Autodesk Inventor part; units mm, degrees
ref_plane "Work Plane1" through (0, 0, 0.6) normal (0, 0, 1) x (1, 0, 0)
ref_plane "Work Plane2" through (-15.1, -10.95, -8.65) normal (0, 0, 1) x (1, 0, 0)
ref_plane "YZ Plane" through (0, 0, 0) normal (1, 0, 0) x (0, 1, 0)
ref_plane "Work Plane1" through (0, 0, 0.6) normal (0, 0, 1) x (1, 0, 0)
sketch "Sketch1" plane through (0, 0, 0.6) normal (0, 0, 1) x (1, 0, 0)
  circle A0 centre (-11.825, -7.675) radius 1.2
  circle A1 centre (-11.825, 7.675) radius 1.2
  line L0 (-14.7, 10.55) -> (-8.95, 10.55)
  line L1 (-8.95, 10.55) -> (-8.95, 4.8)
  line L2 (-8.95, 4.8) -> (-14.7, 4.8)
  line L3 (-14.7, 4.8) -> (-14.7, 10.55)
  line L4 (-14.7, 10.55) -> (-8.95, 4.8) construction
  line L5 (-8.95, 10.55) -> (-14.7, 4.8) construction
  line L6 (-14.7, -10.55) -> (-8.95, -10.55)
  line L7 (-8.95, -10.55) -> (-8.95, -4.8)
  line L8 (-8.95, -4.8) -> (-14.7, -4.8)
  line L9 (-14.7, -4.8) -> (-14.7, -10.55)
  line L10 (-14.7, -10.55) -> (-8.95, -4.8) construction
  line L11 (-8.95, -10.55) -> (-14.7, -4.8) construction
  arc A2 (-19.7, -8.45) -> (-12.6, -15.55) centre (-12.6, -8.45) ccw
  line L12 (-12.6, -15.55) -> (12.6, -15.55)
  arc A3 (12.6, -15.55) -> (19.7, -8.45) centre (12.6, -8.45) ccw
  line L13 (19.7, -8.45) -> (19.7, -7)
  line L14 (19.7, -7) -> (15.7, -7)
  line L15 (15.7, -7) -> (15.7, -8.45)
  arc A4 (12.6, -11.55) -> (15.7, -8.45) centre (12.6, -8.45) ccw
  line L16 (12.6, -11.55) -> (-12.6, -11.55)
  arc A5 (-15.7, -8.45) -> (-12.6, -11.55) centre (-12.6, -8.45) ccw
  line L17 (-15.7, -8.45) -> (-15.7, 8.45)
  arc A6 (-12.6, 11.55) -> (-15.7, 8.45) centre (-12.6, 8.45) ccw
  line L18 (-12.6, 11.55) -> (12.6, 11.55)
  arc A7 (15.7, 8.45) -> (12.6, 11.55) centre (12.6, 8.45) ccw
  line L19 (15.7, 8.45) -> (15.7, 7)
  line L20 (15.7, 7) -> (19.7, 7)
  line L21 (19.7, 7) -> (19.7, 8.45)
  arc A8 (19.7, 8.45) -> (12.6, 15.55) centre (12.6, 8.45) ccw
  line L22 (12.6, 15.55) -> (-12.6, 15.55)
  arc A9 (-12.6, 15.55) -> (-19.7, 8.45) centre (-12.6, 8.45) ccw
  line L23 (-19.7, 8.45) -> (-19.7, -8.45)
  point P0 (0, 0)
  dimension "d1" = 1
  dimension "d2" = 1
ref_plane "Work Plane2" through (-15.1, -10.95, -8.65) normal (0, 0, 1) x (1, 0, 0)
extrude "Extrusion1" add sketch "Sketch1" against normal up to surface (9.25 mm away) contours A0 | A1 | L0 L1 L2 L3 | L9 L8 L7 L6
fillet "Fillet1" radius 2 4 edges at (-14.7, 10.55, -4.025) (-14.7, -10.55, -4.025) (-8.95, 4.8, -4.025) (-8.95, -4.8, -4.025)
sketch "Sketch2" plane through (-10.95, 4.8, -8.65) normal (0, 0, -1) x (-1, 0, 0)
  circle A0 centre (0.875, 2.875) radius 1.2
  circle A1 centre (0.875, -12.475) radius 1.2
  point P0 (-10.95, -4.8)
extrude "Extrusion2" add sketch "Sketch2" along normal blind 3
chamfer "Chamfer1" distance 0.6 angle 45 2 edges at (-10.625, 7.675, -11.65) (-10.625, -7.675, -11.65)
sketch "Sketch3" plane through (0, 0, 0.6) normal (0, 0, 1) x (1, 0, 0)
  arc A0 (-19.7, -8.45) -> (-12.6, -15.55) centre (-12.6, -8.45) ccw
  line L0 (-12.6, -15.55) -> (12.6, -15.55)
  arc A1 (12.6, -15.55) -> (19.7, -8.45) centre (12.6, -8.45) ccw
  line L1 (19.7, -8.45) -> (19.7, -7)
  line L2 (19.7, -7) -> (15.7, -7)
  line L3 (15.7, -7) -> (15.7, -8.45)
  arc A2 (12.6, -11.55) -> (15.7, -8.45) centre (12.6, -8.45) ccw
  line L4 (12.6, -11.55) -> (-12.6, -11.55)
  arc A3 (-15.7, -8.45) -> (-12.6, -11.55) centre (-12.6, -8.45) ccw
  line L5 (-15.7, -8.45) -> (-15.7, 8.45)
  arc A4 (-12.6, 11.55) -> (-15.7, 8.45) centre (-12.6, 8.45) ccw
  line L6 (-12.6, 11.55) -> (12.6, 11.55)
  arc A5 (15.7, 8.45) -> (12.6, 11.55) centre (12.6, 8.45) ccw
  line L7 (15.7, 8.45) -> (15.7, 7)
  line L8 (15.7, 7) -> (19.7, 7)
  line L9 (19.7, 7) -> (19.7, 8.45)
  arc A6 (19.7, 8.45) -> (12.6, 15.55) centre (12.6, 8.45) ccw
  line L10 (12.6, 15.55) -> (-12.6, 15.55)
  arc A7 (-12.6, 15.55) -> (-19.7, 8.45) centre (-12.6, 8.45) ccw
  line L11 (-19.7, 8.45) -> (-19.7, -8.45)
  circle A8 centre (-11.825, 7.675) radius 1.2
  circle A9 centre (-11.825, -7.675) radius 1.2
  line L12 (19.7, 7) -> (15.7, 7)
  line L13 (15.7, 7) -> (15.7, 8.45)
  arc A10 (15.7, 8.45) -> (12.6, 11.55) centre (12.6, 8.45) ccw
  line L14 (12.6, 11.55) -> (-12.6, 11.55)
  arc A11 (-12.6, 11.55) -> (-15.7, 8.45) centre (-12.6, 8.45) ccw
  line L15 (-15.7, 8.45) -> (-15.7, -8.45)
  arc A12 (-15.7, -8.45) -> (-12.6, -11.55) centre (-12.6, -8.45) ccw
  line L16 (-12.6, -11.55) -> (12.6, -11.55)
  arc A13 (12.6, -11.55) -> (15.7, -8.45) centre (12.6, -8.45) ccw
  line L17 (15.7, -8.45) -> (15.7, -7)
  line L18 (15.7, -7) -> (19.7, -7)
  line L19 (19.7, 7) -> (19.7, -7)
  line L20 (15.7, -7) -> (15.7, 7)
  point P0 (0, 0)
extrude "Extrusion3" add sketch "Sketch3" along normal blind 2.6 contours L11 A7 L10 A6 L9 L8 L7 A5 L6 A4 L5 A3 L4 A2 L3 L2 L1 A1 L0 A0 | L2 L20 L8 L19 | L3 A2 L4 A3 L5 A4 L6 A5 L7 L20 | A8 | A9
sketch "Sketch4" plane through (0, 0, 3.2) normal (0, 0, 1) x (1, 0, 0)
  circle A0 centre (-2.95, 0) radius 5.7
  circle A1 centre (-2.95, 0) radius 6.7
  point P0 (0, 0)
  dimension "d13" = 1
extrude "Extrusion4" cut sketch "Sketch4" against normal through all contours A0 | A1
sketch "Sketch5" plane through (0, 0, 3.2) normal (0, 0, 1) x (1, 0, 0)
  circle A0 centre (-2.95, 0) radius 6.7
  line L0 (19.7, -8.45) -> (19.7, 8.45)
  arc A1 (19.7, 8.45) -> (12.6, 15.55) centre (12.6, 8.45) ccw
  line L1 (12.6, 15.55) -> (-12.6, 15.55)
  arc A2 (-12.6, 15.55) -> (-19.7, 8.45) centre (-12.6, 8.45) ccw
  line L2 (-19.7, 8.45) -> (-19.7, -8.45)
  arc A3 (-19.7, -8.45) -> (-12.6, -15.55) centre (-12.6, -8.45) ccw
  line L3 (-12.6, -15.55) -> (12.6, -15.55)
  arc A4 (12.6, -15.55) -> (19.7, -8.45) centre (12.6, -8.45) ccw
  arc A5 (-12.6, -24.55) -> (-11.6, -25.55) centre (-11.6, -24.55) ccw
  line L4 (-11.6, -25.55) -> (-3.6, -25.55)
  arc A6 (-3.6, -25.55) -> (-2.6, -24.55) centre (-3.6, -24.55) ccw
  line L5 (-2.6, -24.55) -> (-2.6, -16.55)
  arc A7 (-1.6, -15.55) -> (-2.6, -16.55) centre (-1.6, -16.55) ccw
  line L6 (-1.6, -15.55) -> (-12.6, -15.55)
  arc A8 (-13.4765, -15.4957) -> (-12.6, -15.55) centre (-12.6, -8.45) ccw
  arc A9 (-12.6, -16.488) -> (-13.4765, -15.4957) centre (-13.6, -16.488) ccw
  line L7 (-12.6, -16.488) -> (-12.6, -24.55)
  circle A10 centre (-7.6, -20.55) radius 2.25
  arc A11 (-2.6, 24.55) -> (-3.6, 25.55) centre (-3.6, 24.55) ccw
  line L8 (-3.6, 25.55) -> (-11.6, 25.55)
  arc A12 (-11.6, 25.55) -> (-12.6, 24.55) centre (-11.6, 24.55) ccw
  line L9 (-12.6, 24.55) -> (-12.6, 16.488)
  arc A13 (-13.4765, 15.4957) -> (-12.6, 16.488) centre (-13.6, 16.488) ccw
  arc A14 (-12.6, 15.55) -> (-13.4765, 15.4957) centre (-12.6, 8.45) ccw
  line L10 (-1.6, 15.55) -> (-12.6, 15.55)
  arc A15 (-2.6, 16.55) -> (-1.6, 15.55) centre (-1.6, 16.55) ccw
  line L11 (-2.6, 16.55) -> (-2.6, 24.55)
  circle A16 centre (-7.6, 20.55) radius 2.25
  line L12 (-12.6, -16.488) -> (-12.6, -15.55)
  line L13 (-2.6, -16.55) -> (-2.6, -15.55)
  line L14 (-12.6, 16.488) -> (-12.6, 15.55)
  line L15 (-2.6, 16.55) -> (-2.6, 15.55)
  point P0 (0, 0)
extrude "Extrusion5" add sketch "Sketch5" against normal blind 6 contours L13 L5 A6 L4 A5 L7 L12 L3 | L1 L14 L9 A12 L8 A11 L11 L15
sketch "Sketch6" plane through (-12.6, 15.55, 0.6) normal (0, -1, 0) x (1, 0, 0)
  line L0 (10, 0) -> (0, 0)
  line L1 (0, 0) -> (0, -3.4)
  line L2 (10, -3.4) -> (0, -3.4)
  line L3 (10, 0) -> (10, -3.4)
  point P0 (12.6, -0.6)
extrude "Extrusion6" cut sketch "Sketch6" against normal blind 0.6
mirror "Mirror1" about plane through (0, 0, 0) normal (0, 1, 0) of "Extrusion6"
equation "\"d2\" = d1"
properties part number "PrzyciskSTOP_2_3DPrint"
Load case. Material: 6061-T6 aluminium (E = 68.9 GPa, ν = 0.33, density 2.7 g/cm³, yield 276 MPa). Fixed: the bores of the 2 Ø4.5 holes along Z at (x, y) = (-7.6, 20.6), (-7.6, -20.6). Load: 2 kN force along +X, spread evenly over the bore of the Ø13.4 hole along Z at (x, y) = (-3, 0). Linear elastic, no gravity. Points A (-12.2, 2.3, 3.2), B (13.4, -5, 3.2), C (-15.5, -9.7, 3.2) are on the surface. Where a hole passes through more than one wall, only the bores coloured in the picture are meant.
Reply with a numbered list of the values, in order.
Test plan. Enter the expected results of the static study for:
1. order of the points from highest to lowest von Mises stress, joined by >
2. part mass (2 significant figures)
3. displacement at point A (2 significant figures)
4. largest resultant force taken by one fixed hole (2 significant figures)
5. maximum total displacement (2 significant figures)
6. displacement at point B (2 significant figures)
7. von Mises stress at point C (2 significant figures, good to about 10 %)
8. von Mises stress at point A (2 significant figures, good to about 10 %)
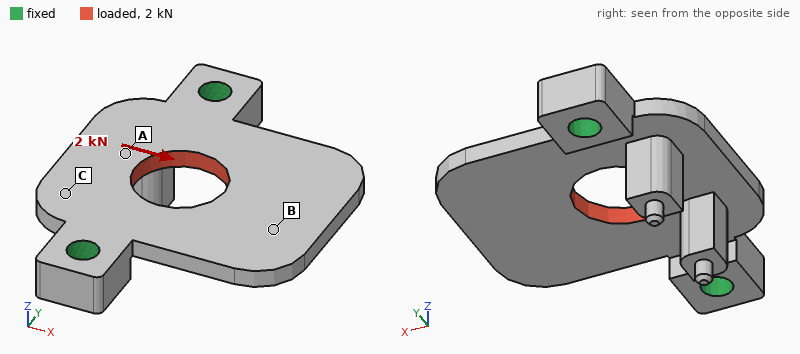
1. C > A > B
2. 12 g
3. 19 µm
4. 1.0 kN
5. 20 µm
6. 16 µm
7. 29 MPa
8. 22 MPa
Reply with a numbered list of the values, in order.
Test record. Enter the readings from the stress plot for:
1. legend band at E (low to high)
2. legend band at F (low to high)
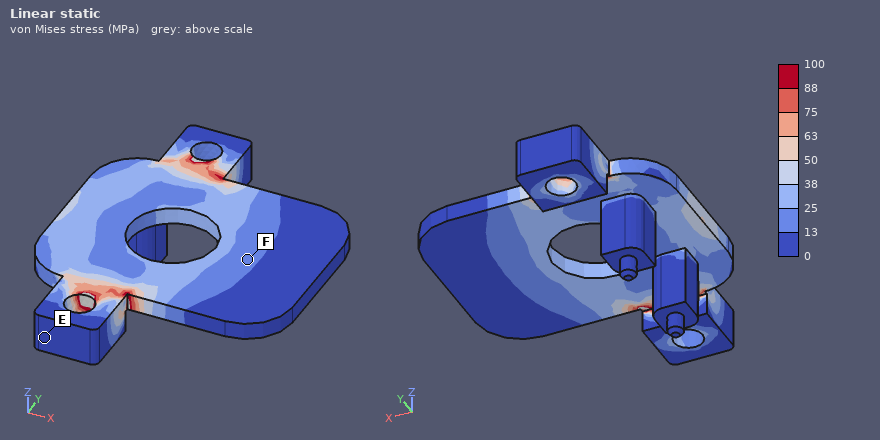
1. 0 to 13 MPa
2. 13 to 25 MPa
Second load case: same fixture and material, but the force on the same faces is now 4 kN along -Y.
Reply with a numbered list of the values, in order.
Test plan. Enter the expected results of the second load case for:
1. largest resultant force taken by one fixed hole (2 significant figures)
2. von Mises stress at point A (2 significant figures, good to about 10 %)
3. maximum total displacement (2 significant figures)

1. 2.1 kN
2. 20 MPa
3. 30 µm
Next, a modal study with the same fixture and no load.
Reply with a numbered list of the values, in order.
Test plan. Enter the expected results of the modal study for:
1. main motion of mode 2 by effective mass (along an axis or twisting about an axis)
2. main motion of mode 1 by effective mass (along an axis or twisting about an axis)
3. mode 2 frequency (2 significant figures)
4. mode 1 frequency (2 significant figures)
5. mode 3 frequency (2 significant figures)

1. along Z
2. along Z
3. 6400 Hz
4. 2300 Hz
5. 6800 Hz
